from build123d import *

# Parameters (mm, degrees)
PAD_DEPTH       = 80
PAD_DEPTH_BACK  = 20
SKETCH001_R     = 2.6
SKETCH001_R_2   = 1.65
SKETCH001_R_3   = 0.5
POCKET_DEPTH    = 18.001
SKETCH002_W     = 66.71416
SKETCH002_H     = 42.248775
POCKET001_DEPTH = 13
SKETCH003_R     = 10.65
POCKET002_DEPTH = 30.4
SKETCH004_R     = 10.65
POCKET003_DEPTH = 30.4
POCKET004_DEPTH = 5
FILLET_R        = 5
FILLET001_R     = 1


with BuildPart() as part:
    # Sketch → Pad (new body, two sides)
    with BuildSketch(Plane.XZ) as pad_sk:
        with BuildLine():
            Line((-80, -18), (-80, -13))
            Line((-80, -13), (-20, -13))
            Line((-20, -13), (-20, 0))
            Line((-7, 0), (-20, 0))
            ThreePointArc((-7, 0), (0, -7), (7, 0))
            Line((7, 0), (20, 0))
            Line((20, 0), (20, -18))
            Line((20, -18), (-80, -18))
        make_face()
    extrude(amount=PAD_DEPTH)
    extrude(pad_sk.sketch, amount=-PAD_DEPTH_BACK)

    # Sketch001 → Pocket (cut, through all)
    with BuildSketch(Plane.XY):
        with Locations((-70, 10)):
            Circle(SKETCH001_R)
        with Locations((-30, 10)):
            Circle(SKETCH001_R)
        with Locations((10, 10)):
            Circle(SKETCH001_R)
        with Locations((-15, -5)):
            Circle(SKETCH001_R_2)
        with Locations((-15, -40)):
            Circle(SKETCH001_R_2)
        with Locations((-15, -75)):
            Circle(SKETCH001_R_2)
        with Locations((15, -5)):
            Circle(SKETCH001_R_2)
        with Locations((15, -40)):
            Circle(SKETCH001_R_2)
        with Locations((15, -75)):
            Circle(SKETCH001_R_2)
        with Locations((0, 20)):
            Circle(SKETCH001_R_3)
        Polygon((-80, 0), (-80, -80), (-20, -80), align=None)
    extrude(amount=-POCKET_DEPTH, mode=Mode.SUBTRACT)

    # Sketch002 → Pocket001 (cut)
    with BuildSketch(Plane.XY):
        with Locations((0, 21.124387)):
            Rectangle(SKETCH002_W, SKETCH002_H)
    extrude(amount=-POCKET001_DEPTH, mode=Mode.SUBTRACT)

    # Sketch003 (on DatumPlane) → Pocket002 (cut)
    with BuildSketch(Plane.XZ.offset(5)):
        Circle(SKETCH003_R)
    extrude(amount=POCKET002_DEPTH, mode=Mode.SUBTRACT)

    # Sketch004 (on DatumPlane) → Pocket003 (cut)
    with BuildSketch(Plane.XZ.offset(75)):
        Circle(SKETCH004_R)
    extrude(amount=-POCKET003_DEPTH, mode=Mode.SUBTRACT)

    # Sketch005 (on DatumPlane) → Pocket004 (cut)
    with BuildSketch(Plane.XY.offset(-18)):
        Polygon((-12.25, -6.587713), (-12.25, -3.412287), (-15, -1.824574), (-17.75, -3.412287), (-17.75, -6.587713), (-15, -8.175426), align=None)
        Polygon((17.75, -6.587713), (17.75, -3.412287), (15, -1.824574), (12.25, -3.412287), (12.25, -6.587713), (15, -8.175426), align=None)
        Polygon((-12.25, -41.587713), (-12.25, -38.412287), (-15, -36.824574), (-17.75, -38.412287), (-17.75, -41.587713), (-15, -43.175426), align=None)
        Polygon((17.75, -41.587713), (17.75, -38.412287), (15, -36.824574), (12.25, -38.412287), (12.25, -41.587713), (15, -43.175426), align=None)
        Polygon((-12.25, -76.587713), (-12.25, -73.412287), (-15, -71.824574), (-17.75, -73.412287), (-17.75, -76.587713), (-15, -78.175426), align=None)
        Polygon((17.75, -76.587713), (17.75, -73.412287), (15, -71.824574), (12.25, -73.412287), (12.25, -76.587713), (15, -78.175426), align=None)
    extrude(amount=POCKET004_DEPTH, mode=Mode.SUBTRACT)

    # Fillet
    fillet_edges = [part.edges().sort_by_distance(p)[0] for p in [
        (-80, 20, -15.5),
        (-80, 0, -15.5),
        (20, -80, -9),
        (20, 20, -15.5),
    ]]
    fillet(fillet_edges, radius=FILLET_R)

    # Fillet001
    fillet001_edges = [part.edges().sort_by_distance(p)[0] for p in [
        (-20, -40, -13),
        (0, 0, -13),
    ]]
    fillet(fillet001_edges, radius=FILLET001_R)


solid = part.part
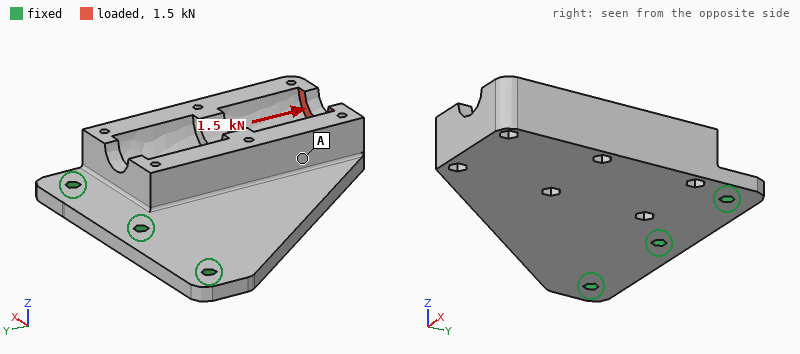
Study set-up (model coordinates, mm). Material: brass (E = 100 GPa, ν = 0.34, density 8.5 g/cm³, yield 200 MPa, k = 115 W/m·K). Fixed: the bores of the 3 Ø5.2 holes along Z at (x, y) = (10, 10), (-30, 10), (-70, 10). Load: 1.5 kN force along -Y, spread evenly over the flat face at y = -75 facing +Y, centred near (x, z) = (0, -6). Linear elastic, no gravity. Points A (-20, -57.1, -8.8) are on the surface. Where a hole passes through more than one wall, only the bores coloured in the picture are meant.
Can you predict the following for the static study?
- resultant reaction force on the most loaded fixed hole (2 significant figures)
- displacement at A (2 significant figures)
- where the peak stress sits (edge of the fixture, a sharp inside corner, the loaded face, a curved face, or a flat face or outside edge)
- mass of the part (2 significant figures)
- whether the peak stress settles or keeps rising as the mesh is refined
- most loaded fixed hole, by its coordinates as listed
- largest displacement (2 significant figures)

1.0 kN
0.17 mm
edge of the fixture
560 g
keeps rising
(10, 10)
0.26 mm
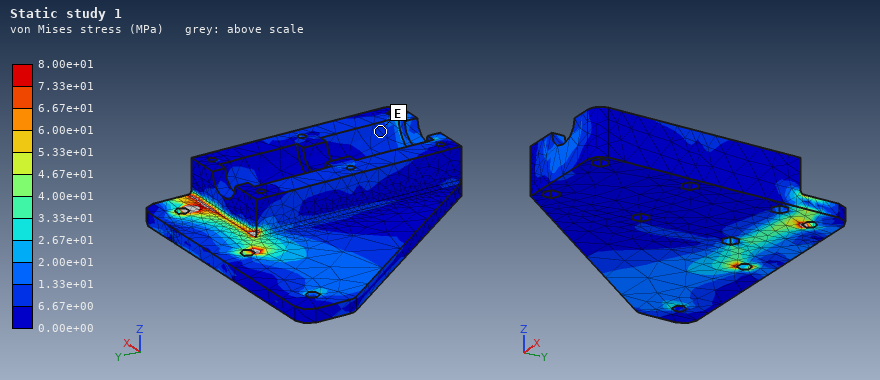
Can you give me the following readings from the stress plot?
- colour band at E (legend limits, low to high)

6.67e+00 to 1.33e+01 MPa
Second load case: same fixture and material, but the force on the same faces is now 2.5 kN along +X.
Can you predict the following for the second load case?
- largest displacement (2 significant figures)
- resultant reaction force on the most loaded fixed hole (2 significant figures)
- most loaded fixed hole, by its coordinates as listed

0.13 mm
3.3 kN
(10, 10)
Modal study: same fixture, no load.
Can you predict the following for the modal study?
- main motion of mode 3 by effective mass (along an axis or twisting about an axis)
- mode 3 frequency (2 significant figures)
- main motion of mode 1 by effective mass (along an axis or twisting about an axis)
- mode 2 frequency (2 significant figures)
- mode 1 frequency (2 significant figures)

along X
3200 Hz
along Z
1800 Hz
350 Hz
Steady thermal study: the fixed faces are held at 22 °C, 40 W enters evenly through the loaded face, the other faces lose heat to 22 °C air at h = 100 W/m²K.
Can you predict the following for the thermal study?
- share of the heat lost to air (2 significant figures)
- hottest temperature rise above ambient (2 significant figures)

66 %
45 K
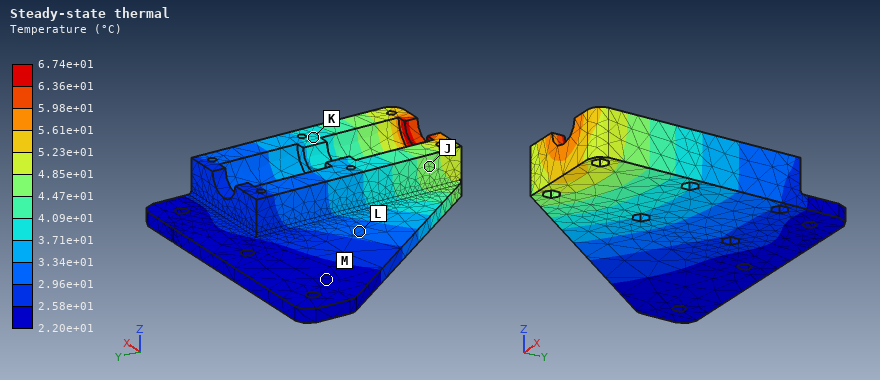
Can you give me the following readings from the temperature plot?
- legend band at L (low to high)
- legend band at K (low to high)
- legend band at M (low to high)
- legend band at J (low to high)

2.96e+01 to 3.34e+01 °C
3.71e+01 to 4.09e+01 °C
2.20e+01 to 2.58e+01 °C
4.47e+01 to 4.85e+01 °C
